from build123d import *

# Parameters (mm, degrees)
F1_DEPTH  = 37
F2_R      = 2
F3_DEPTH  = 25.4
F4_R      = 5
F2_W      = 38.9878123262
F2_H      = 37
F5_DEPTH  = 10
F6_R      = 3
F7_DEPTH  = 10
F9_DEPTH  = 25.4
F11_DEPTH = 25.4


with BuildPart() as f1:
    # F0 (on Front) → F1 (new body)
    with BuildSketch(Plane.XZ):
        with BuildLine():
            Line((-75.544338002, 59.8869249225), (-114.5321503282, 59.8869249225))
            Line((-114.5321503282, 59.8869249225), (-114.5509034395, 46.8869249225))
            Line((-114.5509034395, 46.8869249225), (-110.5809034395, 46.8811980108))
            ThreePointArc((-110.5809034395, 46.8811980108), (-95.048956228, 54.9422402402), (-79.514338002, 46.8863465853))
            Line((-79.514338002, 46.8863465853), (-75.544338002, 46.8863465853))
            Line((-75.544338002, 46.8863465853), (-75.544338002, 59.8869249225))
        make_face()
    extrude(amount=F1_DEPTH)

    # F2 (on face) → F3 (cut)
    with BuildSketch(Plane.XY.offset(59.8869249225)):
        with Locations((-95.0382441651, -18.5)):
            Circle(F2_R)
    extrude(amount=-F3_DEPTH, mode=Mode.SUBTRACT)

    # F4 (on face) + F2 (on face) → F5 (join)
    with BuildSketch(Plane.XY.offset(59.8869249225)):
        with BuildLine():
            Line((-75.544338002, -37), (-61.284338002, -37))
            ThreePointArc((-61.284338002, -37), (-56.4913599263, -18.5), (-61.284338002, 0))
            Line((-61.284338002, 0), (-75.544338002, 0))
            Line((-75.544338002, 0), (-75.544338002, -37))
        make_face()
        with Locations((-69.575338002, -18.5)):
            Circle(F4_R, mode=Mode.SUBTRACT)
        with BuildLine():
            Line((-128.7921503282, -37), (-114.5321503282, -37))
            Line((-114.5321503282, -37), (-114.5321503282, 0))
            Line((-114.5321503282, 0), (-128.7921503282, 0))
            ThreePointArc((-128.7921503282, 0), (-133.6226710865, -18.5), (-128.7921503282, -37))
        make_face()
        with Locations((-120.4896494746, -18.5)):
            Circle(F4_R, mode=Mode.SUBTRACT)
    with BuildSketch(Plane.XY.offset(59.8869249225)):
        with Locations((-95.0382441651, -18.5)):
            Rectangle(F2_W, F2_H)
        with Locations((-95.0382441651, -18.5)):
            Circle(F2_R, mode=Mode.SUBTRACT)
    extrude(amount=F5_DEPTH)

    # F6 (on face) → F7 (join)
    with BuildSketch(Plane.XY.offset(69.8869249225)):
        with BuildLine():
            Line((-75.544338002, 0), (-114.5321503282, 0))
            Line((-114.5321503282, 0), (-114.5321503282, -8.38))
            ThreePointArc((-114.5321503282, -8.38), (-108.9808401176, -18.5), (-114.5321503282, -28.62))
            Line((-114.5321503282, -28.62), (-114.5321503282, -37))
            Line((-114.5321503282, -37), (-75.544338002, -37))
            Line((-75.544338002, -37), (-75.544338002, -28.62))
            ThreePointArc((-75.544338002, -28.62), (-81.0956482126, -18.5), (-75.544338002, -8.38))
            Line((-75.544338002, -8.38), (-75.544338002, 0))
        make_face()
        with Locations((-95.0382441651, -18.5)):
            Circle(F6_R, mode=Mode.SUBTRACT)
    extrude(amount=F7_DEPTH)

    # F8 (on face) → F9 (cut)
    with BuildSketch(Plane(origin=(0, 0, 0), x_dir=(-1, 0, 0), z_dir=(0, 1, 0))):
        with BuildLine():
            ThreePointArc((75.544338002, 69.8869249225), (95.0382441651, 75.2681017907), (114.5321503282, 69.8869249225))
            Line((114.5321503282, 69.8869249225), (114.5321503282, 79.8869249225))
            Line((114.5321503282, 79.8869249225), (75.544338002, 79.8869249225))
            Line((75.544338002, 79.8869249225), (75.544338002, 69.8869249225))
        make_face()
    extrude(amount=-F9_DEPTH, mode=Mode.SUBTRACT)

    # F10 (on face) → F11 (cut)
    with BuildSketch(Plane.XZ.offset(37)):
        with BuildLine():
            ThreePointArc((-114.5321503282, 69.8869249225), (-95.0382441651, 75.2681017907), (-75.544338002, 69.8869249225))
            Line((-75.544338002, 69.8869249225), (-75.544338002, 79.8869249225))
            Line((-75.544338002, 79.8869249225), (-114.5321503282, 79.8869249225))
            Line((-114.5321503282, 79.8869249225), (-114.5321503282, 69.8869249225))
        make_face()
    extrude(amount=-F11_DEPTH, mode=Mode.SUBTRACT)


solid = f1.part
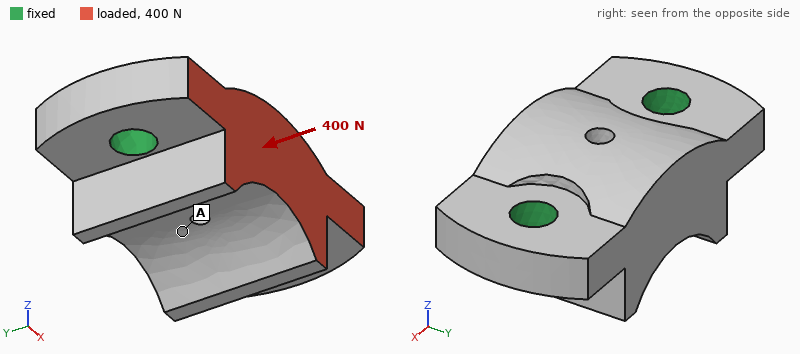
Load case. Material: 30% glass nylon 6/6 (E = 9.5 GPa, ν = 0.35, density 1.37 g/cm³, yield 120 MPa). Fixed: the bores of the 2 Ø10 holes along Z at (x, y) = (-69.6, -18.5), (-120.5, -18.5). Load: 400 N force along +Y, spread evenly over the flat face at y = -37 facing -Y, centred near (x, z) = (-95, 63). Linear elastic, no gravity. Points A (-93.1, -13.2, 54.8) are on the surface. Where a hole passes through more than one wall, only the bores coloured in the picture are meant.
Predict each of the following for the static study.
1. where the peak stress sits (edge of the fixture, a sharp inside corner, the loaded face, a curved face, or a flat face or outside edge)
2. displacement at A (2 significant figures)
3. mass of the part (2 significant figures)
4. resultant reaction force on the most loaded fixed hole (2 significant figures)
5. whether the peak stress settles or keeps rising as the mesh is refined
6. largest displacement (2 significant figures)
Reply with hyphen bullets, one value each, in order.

- edge of the fixture
- 2.2 µm
- 59 g
- 200 N
- keeps rising
- 3.4 µm
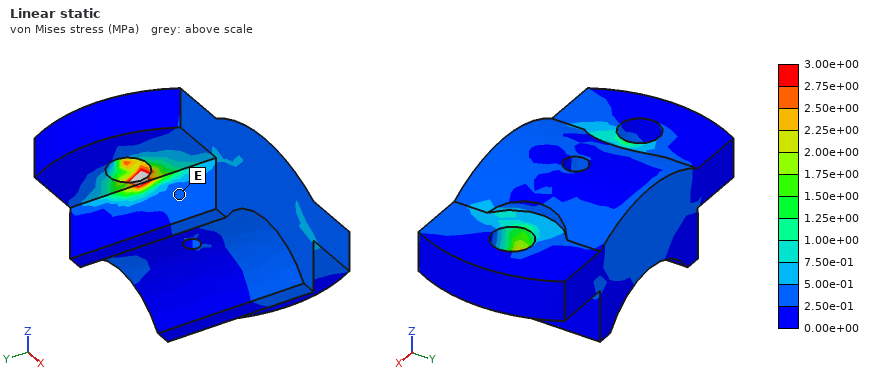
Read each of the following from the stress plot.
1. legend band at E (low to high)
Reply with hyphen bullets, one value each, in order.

- 2.50e-01 to 5.00e-01 MPa
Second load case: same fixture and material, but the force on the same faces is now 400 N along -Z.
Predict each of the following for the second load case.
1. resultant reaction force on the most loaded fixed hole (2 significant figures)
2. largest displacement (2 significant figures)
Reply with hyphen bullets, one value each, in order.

- 200 N
- 18 µm
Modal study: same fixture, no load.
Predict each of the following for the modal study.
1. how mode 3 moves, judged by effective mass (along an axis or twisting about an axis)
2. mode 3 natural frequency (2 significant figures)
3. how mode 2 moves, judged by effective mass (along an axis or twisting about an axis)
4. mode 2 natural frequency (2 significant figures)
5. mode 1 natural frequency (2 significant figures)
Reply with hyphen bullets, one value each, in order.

- along Y
- 11 kHz
- along Z
- 8400 Hz
- 6100 Hz
